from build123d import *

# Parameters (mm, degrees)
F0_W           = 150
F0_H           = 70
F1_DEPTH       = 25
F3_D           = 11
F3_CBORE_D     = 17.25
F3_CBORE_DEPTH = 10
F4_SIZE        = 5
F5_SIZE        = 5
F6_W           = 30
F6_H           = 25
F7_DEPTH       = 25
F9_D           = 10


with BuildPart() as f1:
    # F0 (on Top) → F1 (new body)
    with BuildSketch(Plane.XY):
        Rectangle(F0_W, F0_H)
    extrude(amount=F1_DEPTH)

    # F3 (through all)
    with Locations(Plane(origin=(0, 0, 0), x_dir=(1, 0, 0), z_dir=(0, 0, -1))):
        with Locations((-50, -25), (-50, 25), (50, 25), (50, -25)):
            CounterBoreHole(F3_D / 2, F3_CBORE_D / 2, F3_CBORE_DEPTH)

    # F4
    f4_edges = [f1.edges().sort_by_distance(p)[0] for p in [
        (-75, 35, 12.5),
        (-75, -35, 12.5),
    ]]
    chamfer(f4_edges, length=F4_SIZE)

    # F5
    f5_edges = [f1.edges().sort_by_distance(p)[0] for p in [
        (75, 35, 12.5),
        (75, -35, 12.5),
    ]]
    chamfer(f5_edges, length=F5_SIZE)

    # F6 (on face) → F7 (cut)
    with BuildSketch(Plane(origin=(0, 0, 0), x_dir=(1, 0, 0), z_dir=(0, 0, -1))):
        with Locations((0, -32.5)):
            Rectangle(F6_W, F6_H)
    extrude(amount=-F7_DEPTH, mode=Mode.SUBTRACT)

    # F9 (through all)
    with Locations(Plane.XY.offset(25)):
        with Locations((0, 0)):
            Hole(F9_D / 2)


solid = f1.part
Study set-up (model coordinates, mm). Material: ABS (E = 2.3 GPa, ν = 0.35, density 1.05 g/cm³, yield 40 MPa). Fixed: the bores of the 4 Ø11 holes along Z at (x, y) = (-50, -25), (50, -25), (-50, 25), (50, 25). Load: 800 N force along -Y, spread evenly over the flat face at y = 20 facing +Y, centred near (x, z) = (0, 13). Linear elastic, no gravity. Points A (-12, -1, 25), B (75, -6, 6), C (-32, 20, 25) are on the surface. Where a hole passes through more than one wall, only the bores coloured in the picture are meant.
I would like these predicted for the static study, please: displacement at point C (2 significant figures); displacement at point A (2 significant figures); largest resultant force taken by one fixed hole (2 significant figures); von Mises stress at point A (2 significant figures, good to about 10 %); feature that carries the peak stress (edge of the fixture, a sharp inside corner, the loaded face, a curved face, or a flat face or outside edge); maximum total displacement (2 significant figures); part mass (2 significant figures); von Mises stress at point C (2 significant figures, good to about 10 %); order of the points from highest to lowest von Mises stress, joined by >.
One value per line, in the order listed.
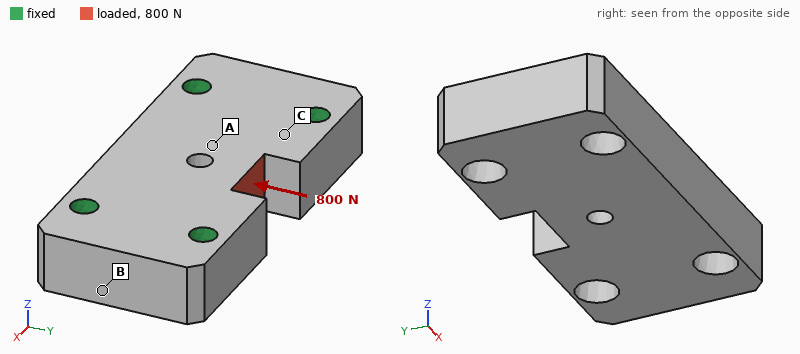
7.3 µm
17 µm
280 N
0.76 MPa
edge of the fixture
28 µm
240 g
0.50 MPa
A > C > B
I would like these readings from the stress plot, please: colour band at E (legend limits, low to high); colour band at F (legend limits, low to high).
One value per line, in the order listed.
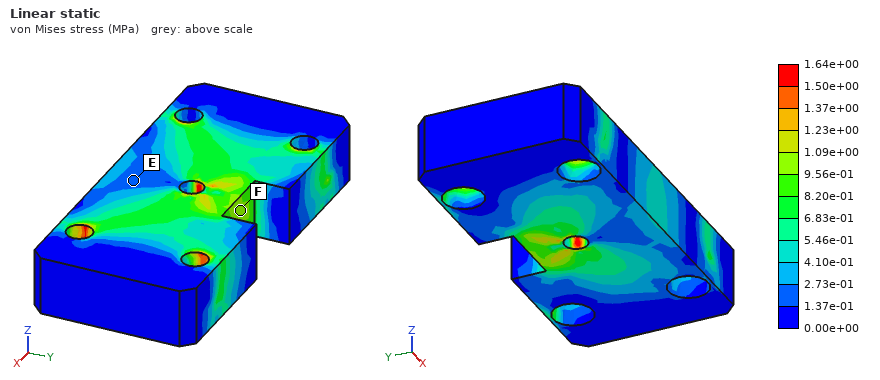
1.37e-01 to 2.73e-01 MPa
9.56e-01 to 1.09e+00 MPa
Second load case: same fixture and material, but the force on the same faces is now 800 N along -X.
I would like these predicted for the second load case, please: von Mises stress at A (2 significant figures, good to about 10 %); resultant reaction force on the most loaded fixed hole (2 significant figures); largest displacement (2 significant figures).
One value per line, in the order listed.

0.29 MPa
230 N
20 µm
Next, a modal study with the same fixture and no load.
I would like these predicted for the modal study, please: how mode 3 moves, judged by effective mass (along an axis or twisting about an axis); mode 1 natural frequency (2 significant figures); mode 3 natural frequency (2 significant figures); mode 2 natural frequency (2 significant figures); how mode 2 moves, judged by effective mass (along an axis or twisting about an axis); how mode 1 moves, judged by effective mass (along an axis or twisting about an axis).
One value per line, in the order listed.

along Y
2300 Hz
3800 Hz
3600 Hz
twisting about X
along Z
